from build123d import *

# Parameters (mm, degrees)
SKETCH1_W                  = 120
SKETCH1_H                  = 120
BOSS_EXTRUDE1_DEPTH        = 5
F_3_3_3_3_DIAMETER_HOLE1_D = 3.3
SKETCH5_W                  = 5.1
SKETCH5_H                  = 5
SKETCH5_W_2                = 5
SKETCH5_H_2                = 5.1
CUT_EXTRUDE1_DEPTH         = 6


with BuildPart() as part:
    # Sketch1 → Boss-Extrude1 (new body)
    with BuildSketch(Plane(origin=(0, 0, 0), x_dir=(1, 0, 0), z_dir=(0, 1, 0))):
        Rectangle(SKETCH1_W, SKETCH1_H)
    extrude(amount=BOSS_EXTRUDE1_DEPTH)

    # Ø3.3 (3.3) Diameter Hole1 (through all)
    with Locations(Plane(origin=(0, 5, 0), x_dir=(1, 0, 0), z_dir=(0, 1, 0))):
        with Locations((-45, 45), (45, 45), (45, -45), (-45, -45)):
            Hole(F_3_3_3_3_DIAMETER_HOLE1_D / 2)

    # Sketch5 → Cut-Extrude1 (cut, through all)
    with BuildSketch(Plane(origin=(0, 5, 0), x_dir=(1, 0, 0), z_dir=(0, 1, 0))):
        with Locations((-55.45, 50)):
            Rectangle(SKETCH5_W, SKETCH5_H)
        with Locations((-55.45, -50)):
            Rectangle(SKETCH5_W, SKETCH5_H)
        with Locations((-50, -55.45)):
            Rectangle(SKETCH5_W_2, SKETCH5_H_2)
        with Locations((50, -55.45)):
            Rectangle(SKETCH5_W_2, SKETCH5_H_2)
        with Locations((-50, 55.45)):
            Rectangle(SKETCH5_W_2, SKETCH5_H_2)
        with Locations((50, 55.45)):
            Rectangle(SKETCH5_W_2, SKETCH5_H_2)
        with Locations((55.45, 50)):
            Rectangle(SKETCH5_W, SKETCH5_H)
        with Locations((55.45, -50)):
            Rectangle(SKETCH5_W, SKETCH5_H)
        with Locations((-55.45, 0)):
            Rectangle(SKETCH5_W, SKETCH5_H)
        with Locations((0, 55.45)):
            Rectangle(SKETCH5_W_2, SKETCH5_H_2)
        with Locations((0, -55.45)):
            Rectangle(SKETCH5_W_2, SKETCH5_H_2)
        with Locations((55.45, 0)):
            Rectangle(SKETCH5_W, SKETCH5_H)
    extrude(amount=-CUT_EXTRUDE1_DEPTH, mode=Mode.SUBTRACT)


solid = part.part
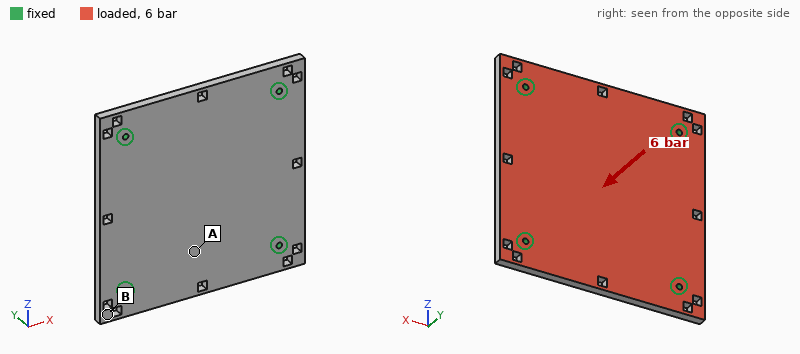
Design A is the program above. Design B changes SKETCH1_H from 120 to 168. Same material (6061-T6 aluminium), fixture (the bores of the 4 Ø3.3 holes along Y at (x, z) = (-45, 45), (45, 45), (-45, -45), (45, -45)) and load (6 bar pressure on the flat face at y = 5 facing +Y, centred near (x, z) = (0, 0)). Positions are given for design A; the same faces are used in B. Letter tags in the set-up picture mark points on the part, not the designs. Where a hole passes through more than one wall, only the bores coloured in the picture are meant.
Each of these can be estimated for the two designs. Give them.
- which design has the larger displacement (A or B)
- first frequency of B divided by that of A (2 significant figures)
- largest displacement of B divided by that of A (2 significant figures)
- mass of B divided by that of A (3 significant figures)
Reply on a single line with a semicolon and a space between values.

B; 0.82; 1.4; 1.41
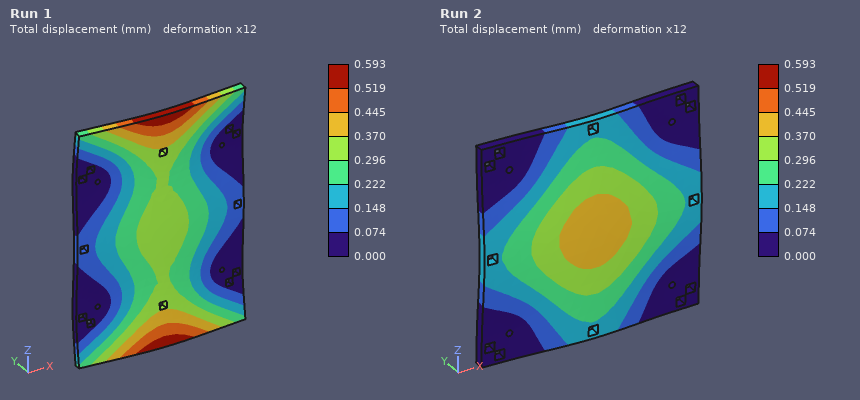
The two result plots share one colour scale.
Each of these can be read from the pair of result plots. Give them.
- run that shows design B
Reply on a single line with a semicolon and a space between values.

Run 1
